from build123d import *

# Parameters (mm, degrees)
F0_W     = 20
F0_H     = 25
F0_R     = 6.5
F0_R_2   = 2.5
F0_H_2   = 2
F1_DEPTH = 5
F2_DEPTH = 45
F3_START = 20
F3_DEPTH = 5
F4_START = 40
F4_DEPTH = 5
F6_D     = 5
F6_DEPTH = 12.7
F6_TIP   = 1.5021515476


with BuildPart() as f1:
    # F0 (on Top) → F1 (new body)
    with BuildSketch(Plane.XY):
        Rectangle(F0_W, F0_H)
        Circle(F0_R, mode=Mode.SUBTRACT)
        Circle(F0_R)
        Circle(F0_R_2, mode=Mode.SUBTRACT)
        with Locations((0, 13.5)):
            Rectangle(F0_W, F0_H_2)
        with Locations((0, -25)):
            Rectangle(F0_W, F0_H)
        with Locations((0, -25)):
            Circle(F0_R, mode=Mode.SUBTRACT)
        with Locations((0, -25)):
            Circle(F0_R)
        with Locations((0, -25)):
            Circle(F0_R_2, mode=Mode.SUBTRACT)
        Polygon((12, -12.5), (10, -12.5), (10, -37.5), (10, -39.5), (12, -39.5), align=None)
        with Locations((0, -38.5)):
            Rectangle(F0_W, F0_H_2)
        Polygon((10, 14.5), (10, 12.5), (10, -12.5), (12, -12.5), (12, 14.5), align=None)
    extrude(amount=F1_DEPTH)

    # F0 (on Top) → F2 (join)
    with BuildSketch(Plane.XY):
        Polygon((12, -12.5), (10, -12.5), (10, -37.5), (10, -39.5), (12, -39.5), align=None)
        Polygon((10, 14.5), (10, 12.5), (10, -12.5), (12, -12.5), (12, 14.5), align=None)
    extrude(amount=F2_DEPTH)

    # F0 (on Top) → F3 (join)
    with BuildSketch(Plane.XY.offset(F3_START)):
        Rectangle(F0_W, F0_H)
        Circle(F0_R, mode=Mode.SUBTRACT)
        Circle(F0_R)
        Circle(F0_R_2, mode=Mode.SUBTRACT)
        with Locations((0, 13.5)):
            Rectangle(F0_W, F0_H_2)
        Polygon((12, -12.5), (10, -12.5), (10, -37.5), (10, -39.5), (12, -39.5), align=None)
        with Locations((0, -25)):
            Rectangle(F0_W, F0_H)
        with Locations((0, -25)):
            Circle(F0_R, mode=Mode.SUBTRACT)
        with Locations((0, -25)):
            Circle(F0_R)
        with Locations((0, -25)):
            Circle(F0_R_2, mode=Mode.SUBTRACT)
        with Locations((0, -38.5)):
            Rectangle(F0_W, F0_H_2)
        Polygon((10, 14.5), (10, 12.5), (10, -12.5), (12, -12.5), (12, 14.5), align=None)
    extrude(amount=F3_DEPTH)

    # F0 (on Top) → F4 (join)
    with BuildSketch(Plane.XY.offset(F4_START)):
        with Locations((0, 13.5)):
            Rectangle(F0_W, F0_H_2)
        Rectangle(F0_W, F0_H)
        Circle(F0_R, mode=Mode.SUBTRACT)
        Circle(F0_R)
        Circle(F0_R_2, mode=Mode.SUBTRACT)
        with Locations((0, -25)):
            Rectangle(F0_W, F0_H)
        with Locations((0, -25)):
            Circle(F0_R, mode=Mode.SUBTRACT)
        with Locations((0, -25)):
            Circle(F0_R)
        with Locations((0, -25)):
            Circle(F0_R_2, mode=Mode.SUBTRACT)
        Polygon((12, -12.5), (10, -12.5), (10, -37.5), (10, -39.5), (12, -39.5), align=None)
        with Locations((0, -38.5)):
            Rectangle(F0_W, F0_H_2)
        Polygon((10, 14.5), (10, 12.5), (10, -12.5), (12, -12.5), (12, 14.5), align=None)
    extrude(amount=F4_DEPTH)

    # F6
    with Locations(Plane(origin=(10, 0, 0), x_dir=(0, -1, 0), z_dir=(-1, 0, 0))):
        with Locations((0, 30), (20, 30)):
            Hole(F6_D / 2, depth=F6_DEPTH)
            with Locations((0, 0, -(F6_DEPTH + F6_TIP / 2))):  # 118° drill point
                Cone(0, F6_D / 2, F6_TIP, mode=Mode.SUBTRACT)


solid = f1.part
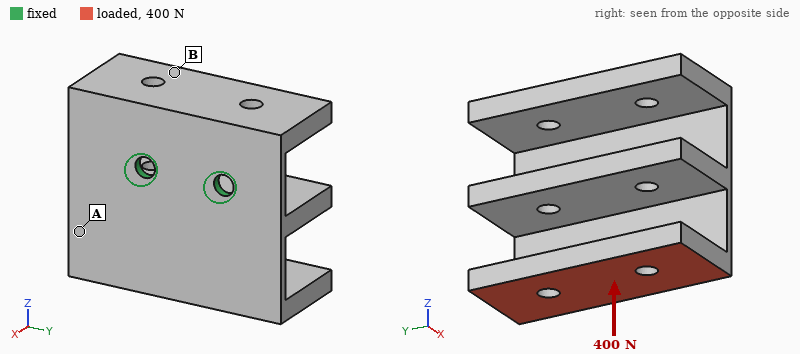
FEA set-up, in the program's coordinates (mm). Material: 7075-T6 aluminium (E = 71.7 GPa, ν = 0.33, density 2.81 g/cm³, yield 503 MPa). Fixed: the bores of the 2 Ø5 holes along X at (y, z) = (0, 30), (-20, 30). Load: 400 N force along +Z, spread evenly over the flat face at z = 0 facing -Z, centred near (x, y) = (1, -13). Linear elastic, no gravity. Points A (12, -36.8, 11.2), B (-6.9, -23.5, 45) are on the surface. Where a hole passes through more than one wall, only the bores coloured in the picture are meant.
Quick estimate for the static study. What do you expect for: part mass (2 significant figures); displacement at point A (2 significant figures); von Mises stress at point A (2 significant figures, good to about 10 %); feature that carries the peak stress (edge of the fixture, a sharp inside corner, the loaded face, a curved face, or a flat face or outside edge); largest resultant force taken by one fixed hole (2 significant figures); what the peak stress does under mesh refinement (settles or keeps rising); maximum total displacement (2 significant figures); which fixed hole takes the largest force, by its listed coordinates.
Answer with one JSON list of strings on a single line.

["57 g", "0.19 mm", "100 MPa", "edge of the fixture", "240 N", "keeps rising", "0.84 mm", "(-20, 30)"]
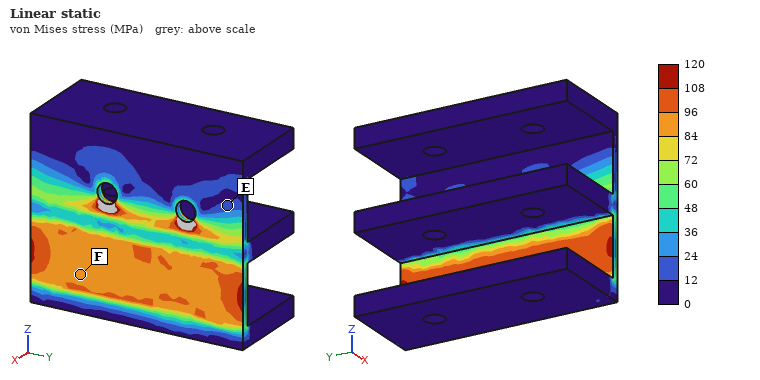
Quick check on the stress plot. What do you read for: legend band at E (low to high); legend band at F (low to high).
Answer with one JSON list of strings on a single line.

["12 to 24 MPa", "84 to 96 MPa"]
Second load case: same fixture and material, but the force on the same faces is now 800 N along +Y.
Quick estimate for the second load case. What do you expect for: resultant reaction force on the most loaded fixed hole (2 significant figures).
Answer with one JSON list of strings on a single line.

["1.2 kN"]
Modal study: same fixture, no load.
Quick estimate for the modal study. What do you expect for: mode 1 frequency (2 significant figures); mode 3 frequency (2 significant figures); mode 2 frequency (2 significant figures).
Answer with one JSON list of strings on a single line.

["710 Hz", "1900 Hz", "1500 Hz"]
